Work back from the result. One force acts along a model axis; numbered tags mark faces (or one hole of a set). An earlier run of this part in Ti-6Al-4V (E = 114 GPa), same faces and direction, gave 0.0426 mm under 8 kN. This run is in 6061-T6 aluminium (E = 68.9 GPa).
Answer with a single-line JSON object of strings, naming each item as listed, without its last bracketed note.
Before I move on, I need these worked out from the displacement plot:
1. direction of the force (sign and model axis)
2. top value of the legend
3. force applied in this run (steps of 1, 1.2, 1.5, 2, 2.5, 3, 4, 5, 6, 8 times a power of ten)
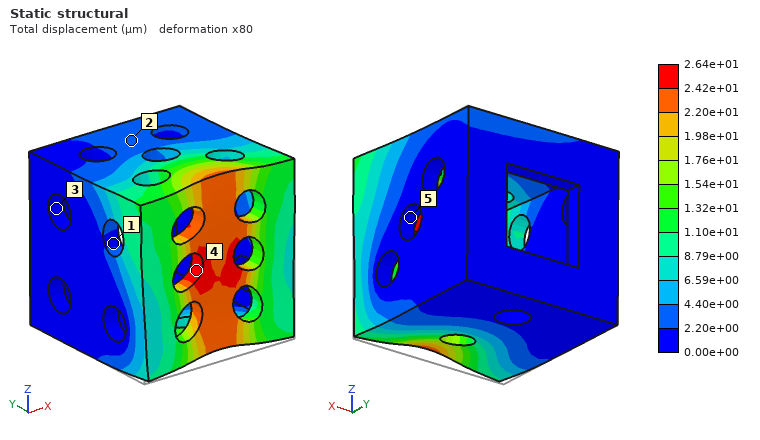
{"direction of the force": "+Z", "top value of the legend": "2.64e+01 µm", "force applied in this run": "3 kN"}
